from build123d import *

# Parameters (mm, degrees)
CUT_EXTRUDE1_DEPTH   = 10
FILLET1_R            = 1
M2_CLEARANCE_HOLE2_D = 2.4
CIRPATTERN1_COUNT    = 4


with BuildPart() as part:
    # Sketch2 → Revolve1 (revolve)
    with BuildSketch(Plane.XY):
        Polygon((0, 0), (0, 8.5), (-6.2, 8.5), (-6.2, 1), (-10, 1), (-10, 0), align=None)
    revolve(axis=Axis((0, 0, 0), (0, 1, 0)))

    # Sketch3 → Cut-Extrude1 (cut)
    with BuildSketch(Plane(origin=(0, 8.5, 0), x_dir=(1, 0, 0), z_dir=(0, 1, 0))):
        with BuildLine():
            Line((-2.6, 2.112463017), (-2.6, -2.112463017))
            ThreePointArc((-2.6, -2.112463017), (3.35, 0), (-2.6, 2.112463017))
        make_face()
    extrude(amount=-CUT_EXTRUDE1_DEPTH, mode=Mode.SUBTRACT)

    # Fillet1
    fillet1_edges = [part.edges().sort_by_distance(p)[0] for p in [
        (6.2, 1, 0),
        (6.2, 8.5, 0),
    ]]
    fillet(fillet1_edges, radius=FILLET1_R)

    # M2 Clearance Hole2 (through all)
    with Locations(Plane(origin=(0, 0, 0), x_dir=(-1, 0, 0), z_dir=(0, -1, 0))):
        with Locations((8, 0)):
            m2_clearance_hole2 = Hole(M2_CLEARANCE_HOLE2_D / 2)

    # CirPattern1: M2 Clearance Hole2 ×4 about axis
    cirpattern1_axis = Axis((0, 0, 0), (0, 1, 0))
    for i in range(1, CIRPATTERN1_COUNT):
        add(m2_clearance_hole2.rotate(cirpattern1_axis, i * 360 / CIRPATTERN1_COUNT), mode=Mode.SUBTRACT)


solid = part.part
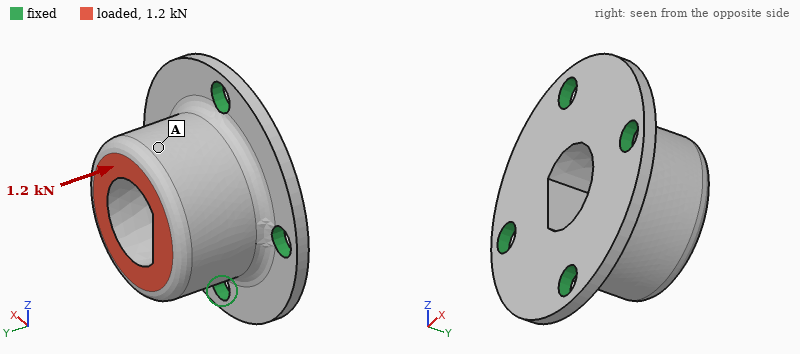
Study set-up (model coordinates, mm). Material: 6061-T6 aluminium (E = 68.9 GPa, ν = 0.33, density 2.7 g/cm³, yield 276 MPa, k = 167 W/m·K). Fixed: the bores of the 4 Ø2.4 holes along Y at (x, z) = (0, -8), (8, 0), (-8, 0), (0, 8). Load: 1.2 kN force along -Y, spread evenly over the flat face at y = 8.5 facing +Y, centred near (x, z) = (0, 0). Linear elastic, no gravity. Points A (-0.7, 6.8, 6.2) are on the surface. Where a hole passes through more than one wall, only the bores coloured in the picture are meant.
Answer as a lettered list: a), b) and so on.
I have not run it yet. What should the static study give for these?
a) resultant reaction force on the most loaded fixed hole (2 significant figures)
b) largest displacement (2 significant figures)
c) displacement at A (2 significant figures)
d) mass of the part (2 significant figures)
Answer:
a) 360 N
b) 7.6 µm
c) 6.4 µm
d) 2.5 g
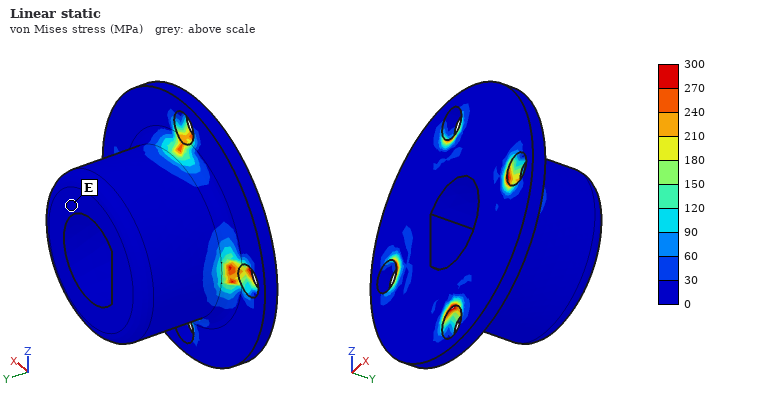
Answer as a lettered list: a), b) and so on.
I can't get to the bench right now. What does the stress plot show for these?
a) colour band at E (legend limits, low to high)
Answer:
a) 0 to 30 MPa
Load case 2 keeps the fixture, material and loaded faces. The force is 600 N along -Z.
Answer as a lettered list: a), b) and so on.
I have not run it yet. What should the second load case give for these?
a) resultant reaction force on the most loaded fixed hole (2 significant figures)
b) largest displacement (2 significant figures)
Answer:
a) 410 N
b) 13 µm
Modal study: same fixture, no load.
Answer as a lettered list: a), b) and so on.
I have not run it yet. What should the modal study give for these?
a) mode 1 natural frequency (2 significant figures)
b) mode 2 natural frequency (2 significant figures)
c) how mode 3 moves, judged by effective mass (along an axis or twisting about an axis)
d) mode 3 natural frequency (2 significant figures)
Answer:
a) 39 kHz
b) 39 kHz
c) along Y
d) 47 kHz
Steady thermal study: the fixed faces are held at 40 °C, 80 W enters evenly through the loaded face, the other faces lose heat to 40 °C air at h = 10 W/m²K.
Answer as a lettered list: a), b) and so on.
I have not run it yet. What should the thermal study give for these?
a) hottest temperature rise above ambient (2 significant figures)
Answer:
a) 78 K
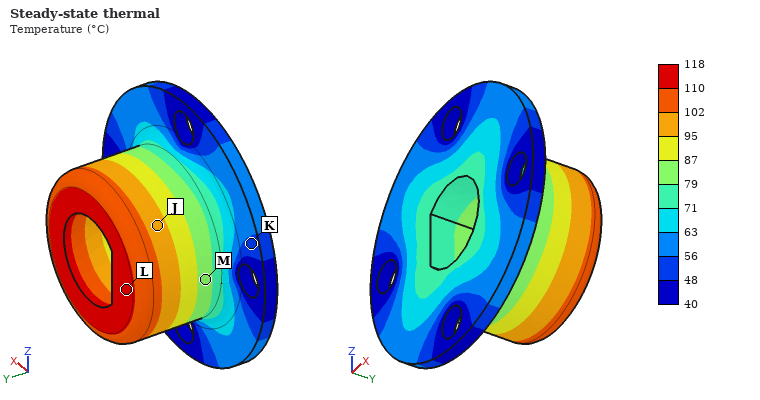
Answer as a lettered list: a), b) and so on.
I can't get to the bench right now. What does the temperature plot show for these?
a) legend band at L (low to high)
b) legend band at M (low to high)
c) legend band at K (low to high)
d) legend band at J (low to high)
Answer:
a) 110 to 118 °C
b) 79 to 87 °C
c) 48 to 56 °C
d) 95 to 102 °C
